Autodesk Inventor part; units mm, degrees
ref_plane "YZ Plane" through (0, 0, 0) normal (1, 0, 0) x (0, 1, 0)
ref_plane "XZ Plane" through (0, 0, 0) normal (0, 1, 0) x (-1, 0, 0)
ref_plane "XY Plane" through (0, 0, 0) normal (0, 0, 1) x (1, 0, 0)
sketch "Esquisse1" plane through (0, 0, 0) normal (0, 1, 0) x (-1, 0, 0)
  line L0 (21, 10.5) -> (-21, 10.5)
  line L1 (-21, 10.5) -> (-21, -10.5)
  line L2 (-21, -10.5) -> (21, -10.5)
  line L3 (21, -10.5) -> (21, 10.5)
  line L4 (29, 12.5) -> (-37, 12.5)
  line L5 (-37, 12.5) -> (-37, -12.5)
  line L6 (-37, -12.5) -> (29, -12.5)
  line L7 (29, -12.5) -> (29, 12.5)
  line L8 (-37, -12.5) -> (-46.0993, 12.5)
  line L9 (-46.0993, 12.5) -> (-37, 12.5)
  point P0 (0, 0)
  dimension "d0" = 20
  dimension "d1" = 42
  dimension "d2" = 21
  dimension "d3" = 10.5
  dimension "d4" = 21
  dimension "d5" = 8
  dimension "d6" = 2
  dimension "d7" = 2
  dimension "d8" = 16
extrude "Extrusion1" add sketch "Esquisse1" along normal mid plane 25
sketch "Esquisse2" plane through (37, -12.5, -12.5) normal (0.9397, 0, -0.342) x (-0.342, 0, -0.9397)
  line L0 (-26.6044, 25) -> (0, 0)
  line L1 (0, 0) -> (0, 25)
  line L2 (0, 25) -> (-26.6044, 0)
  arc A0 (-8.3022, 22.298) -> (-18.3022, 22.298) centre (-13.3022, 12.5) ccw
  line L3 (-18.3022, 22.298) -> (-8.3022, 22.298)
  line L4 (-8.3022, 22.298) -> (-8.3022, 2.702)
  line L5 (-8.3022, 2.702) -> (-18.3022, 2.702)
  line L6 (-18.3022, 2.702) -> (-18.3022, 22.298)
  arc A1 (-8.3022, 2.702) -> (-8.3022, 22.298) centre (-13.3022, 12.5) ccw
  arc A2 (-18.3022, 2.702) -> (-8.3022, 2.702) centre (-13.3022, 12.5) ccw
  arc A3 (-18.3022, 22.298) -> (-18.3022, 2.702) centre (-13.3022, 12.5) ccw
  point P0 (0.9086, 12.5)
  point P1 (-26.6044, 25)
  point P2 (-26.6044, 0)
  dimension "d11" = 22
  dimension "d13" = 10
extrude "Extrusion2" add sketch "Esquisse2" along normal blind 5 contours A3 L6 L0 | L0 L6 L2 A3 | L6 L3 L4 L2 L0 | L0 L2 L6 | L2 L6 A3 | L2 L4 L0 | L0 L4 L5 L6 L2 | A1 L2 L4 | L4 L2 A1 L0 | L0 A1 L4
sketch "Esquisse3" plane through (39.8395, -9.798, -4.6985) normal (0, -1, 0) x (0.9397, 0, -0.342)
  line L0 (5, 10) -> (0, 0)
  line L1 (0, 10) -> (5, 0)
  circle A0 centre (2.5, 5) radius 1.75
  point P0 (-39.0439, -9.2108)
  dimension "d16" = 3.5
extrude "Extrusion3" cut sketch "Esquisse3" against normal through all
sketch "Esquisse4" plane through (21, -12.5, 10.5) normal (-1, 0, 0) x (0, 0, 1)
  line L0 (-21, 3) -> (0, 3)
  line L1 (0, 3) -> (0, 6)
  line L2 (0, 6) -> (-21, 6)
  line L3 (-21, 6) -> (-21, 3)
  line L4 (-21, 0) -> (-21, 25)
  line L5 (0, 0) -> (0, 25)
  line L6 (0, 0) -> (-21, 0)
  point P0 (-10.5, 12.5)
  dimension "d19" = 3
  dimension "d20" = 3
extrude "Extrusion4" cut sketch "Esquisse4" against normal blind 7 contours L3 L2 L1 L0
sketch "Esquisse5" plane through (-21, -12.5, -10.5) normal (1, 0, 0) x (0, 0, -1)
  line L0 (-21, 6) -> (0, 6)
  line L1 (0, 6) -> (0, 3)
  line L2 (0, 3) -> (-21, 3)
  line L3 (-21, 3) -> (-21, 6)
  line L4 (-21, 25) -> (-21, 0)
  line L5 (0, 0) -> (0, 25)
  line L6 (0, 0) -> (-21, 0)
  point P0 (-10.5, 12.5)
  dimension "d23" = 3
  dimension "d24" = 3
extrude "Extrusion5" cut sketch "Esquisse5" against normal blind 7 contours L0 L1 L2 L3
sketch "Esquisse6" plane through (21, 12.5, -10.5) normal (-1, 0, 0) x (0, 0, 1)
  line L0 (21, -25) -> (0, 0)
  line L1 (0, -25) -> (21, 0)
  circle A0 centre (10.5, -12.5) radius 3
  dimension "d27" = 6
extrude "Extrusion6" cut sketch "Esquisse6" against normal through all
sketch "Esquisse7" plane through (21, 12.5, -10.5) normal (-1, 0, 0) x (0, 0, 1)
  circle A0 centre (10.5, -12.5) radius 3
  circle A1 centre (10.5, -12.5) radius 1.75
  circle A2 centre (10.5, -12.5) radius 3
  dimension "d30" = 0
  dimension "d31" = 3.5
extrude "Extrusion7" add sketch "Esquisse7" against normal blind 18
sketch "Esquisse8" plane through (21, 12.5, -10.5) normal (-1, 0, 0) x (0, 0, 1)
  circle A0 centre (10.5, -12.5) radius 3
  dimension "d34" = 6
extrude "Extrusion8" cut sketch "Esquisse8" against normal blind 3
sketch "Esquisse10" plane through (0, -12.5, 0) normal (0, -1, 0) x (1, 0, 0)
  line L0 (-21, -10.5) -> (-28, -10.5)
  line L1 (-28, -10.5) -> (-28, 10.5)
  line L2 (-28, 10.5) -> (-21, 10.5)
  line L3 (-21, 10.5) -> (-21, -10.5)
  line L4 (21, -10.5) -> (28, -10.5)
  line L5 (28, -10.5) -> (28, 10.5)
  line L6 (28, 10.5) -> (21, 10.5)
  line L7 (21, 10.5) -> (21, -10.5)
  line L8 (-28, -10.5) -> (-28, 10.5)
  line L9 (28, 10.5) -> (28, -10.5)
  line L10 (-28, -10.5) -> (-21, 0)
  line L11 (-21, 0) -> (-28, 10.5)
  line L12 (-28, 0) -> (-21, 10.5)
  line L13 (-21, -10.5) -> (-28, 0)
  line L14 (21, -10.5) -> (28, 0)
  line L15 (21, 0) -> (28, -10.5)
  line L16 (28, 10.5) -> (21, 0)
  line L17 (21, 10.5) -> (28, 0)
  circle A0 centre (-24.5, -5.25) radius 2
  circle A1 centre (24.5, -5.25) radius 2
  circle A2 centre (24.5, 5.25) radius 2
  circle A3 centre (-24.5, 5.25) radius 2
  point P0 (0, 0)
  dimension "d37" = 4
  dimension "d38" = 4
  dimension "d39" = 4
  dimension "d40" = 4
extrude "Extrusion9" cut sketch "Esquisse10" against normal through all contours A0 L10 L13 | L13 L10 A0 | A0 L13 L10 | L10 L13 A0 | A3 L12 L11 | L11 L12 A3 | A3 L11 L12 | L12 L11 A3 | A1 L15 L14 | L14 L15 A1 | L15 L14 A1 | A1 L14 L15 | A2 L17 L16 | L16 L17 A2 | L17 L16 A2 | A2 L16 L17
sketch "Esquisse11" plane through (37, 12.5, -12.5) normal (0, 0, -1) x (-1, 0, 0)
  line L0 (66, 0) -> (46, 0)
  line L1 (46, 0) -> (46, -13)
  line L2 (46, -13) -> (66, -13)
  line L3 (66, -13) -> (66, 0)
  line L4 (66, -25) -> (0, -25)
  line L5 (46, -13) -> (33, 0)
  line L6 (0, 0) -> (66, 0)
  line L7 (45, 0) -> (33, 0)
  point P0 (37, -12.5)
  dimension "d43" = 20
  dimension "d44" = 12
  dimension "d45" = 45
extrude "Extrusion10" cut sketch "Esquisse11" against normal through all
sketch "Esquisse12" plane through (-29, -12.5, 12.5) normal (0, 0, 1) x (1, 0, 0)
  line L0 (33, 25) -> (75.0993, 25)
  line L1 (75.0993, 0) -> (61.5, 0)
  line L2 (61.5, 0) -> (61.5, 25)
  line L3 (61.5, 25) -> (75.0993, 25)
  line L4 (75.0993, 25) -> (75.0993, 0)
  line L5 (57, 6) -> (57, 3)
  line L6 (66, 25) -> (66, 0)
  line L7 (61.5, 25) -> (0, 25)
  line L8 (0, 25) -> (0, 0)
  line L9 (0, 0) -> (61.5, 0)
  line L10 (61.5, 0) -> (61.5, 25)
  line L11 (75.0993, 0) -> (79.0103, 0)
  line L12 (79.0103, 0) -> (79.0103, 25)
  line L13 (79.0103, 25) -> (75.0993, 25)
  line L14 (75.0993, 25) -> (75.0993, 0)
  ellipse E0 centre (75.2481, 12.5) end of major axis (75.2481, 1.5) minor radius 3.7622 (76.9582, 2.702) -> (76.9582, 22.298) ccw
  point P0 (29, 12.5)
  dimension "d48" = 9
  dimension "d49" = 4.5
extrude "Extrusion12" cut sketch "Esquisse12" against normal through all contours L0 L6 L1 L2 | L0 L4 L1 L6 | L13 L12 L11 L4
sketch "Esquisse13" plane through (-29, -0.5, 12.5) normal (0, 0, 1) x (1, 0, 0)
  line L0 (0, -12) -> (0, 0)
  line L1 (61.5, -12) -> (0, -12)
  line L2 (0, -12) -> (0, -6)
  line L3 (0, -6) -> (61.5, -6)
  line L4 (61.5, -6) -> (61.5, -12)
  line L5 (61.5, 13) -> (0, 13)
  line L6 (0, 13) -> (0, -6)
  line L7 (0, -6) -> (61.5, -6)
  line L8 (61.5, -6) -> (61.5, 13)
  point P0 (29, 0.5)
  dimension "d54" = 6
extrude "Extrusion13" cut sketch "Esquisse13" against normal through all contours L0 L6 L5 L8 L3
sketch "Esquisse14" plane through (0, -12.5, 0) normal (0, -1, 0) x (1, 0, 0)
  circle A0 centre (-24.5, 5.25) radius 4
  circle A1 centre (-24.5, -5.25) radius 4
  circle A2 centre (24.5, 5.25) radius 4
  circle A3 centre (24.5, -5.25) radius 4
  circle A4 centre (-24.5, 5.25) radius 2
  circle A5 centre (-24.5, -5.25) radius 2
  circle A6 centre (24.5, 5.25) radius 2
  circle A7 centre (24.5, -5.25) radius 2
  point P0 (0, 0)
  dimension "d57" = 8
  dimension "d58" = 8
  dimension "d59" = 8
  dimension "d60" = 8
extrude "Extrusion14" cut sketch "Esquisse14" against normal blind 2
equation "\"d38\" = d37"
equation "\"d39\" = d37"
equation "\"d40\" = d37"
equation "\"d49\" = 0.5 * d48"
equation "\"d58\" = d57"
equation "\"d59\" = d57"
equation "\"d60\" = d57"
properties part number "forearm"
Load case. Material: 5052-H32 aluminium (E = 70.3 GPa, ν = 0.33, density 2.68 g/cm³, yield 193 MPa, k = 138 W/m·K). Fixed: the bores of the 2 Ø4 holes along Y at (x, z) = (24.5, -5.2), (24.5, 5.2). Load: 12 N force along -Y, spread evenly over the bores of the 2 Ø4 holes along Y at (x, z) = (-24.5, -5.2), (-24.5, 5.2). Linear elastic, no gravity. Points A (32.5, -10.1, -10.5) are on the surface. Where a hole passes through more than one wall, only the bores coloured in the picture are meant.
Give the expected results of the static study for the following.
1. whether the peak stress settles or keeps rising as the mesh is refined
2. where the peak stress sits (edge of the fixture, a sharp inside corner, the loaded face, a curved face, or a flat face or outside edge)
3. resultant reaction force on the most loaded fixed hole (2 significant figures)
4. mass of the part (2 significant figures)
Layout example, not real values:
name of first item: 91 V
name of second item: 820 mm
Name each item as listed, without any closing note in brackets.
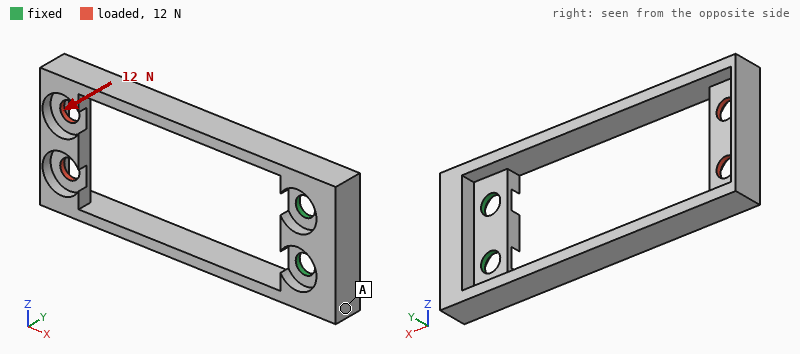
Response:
whether the peak stress settles or keeps rising as the mesh is refined: keeps rising
where the peak stress sits: edge of the fixture
resultant reaction force on the most loaded fixed hole: 6.8 N
mass of the part: 7.0 g
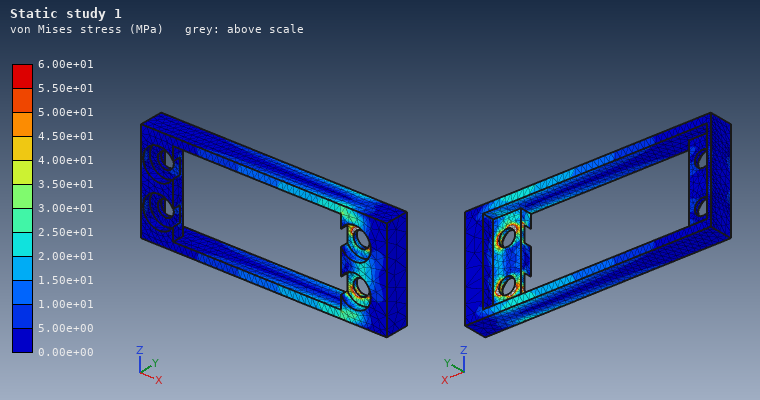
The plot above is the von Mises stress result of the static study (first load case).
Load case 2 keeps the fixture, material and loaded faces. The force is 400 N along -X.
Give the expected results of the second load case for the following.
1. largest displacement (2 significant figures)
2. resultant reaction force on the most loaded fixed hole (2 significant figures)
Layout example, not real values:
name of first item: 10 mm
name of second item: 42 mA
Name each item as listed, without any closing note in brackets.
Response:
largest displacement: 57 µm
resultant reaction force on the most loaded fixed hole: 230 N
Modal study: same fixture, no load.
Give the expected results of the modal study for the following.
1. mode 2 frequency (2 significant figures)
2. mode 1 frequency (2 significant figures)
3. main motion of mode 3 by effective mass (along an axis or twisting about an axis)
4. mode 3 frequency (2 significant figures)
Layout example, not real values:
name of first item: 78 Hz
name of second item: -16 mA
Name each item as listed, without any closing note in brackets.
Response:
mode 2 frequency: 840 Hz
mode 1 frequency: 840 Hz
main motion of mode 3 by effective mass: twisting about X
mode 3 frequency: 1900 Hz
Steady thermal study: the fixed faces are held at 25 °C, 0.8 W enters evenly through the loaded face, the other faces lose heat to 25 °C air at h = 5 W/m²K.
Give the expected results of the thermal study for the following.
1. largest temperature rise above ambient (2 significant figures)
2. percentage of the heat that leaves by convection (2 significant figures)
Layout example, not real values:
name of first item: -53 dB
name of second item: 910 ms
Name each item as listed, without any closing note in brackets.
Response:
largest temperature rise above ambient: 13 K
percentage of the heat that leaves by convection: 11 %
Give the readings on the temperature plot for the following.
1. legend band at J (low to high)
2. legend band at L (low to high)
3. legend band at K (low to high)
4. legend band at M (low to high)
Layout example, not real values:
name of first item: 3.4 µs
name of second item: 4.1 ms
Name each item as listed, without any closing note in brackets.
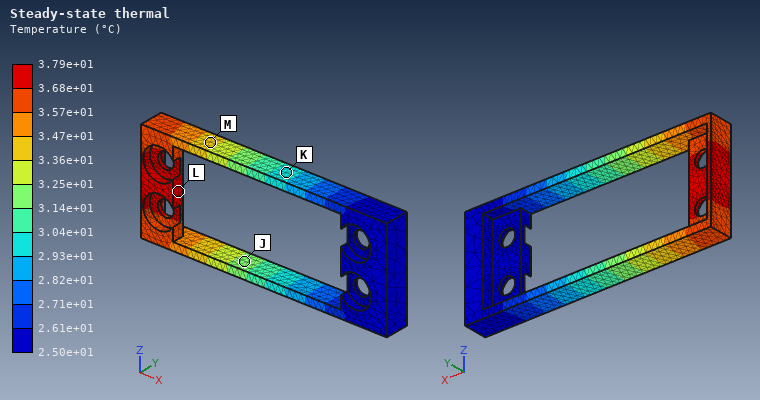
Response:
legend band at J: 3.14e+01 to 3.25e+01 °C
legend band at L: 3.68e+01 to 3.79e+01 °C
legend band at K: 2.93e+01 to 3.04e+01 °C
legend band at M: 3.36e+01 to 3.47e+01 °C
